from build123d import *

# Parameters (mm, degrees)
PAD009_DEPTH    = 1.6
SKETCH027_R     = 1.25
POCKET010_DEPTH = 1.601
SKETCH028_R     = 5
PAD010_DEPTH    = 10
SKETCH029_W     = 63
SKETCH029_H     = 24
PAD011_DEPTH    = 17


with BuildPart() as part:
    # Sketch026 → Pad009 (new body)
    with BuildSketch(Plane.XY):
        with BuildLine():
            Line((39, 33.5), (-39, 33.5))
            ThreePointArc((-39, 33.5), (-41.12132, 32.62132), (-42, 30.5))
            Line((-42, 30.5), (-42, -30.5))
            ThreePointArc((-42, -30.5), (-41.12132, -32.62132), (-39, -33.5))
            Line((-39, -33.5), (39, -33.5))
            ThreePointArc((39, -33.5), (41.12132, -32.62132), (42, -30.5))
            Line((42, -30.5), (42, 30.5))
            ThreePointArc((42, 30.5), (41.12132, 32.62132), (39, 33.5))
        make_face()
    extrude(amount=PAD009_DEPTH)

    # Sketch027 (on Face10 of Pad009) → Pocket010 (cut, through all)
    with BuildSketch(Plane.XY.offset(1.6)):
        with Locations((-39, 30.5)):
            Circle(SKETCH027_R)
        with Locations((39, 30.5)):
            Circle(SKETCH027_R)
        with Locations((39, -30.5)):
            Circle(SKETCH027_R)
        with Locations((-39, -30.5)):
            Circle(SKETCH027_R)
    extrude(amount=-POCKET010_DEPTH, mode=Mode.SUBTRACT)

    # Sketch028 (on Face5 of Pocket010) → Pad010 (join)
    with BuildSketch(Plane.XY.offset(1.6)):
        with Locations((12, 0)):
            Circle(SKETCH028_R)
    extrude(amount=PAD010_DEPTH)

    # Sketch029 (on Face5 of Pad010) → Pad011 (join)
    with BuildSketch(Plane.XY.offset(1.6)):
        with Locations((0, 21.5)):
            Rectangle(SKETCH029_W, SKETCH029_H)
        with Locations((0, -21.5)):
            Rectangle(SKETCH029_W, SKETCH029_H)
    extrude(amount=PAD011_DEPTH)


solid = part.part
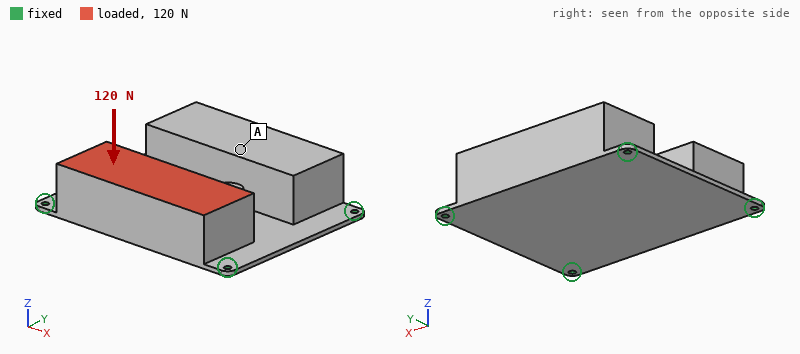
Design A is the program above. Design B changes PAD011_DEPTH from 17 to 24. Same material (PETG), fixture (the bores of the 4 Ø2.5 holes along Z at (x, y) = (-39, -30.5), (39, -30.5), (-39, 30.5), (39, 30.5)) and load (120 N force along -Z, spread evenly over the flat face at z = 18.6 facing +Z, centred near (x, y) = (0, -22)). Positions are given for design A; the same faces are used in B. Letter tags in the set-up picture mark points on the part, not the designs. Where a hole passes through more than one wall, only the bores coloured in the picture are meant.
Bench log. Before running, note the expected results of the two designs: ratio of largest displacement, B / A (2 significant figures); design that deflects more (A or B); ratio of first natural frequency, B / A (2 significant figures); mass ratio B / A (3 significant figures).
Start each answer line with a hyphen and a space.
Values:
- 1.1
- B
- 0.74
- 1.35
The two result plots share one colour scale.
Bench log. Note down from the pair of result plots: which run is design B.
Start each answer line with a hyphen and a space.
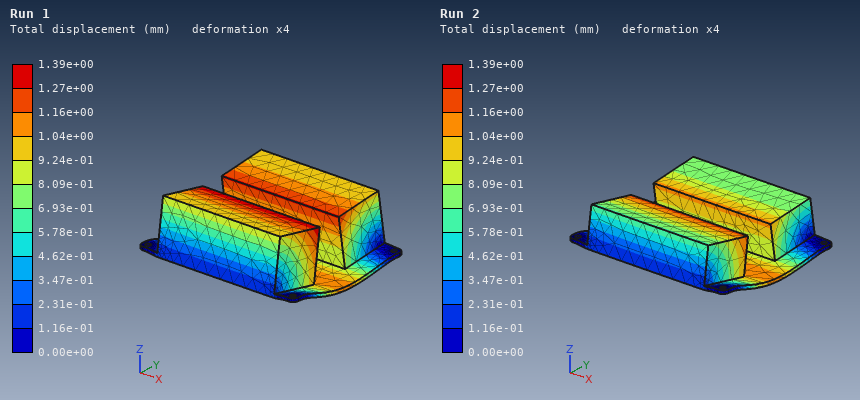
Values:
- Run 1
